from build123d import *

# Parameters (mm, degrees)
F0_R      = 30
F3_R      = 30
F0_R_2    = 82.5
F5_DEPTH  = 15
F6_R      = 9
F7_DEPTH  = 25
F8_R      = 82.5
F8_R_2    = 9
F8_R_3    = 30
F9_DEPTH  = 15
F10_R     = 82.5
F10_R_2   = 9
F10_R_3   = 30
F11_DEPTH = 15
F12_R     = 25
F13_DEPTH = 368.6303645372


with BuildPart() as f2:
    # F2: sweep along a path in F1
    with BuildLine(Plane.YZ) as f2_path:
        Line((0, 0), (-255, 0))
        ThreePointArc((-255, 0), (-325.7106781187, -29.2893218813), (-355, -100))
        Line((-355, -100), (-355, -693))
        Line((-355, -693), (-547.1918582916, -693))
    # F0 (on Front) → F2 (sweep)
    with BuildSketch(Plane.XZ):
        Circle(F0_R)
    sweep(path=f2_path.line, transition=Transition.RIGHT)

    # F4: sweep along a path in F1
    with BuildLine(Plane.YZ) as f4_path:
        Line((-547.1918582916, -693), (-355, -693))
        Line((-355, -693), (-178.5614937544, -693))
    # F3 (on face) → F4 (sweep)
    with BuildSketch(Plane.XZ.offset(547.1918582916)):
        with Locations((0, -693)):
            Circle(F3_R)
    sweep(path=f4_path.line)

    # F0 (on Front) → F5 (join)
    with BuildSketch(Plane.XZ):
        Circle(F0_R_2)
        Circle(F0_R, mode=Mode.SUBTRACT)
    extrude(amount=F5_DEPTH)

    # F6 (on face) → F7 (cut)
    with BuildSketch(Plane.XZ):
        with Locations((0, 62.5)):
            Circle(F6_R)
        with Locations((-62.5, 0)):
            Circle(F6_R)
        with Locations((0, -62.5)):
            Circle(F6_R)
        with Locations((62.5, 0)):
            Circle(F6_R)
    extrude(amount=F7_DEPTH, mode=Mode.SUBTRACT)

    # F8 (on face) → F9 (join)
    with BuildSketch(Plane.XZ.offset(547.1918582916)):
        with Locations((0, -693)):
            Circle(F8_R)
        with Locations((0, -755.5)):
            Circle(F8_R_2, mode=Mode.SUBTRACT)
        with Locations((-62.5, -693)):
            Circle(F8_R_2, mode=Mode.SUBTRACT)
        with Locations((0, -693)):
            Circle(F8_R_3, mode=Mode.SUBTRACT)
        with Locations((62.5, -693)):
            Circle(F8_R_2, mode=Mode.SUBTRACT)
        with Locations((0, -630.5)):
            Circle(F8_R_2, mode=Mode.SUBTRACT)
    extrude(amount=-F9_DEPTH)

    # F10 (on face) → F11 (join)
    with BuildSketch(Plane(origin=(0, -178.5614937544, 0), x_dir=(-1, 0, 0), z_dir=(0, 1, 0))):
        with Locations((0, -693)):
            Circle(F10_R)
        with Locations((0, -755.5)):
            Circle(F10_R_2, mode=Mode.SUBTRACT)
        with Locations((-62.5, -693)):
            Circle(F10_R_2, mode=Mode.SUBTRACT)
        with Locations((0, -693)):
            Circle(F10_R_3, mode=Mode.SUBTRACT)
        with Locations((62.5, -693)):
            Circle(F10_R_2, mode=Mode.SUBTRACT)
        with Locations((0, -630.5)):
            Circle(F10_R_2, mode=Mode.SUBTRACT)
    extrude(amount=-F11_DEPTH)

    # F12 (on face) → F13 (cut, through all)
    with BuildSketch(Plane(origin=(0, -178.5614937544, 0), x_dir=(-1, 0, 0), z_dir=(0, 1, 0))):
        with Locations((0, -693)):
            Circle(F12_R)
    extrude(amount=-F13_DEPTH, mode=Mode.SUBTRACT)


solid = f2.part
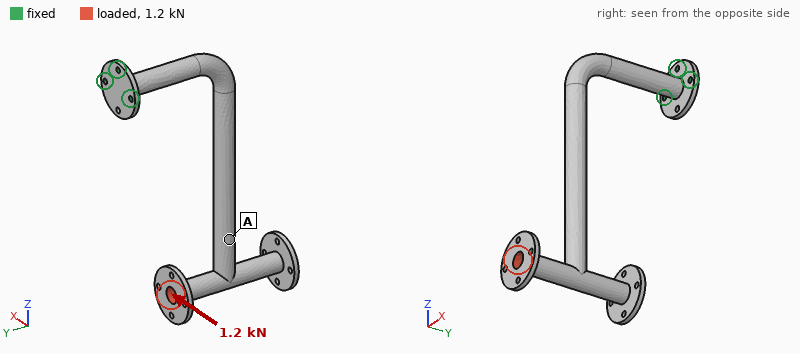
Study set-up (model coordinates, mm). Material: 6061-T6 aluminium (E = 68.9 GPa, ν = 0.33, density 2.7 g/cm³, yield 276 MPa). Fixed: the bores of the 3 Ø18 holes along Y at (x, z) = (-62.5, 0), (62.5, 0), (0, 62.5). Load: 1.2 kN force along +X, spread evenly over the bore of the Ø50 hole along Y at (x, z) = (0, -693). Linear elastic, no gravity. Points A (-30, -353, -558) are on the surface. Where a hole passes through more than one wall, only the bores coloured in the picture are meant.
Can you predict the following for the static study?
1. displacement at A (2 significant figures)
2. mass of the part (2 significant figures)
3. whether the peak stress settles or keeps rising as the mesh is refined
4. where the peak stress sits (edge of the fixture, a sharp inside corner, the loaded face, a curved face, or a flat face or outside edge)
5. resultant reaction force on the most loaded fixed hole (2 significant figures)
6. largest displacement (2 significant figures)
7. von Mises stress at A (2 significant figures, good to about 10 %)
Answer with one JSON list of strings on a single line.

["7.1 mm", "10 kg", "keeps rising", "edge of the fixture", "6.9 kN", "11 mm", "7.9 MPa"]
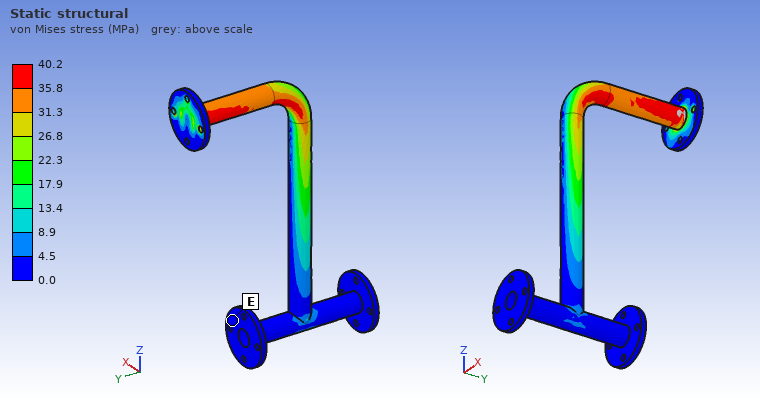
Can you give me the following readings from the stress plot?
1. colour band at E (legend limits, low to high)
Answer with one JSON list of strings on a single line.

["0.0 to 4.5 MPa"]
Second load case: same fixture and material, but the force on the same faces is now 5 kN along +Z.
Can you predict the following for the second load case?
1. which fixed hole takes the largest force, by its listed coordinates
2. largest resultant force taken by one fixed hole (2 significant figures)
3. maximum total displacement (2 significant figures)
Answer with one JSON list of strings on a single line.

["(0, 62.5)", "24 kN", "11 mm"]
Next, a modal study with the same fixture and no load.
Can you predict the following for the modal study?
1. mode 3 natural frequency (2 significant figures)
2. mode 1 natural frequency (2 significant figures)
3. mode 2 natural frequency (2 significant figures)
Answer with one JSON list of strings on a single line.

["110 Hz", "29 Hz", "30 Hz"]
